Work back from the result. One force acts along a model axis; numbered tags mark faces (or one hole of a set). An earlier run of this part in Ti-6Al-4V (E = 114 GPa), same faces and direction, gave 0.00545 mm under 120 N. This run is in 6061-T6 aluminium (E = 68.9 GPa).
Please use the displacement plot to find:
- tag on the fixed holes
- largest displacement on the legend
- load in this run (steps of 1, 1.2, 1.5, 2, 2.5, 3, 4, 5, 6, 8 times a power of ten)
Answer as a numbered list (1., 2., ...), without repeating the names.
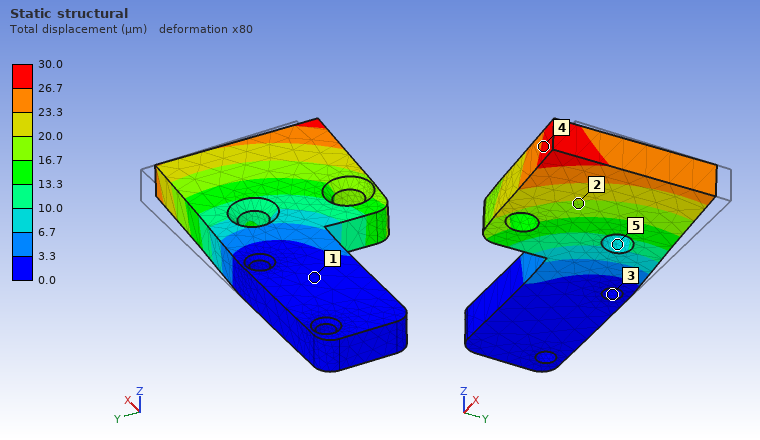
1. 3
2. 30.0 µm
3. 400 N
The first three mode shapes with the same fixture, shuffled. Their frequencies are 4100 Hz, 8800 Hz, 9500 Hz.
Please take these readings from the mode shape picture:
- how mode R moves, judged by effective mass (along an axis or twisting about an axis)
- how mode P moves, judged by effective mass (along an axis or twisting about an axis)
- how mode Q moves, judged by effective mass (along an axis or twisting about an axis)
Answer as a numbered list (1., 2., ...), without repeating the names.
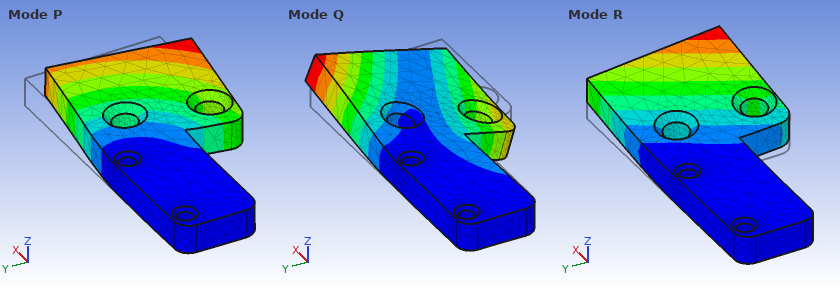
1. along Z
2. along Y
3. twisting about X
